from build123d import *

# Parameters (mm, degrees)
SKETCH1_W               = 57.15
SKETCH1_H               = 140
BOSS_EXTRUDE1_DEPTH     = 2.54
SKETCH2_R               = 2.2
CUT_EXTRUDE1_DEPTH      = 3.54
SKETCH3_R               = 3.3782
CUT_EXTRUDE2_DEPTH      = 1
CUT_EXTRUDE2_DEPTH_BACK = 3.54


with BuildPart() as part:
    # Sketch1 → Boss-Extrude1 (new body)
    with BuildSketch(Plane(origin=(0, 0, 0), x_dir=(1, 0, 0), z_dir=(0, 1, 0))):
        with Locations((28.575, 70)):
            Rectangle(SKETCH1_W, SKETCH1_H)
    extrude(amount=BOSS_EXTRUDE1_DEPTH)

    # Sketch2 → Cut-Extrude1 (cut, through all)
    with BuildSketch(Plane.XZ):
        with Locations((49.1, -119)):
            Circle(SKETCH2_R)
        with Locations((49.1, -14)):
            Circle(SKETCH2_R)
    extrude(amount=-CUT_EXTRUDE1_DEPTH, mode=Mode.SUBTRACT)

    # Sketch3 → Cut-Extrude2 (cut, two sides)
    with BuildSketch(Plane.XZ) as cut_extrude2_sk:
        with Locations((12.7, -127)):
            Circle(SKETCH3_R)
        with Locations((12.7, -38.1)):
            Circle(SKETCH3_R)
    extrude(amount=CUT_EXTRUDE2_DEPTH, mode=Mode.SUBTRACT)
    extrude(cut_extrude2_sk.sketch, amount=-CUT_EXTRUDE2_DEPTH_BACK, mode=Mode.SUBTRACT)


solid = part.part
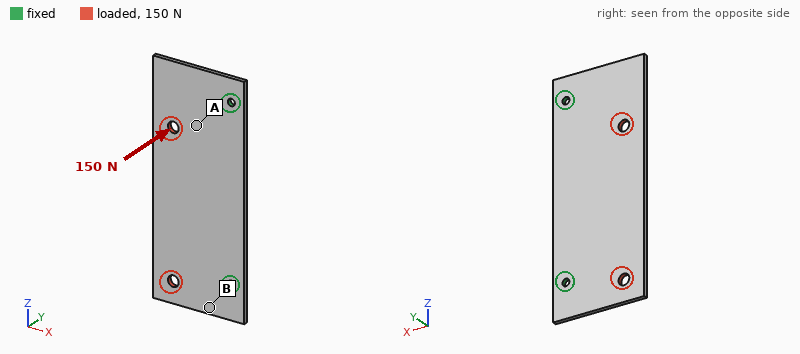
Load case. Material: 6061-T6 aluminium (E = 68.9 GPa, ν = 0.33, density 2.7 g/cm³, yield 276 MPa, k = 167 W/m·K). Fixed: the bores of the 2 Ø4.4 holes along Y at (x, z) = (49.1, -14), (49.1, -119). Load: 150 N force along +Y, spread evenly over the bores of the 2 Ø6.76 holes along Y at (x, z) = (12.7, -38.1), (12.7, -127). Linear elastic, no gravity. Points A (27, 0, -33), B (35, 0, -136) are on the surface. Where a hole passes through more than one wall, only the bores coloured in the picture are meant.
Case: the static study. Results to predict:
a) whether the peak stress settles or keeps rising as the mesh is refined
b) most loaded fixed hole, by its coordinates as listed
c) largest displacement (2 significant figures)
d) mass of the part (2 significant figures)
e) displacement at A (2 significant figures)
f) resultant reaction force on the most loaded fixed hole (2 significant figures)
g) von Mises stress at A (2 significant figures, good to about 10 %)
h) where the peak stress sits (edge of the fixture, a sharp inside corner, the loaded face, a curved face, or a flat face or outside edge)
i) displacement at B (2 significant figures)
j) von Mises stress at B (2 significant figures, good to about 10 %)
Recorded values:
keeps rising
(49.1, -119)
0.56 mm
54 g
0.20 mm
92 N
18 MPa
edge of the fixture
0.084 mm
36 MPa
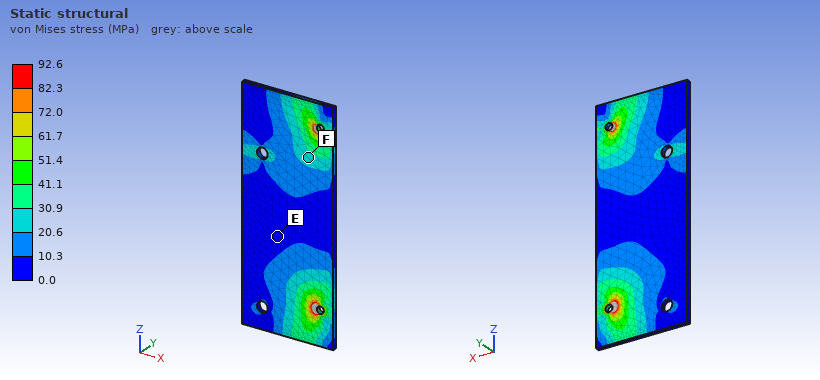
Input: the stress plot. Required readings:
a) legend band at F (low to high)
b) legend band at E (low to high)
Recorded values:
20.6 to 30.9 MPa
0.0 to 10.3 MPa
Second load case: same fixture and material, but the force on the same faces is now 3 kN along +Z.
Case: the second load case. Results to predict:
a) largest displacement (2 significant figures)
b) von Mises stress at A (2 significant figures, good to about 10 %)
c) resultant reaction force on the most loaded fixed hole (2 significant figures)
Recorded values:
42 µm
21 MPa
1.8 kN
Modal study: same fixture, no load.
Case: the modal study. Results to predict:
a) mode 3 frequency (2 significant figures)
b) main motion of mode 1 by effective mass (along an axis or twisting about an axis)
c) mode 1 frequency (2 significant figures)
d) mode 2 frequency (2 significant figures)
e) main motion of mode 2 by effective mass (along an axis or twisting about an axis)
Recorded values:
1200 Hz
along Y
570 Hz
1000 Hz
twisting about X
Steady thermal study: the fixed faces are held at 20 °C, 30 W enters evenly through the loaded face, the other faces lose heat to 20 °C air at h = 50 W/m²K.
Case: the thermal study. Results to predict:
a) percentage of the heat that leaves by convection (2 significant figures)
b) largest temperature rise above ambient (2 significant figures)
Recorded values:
40 %
35 K
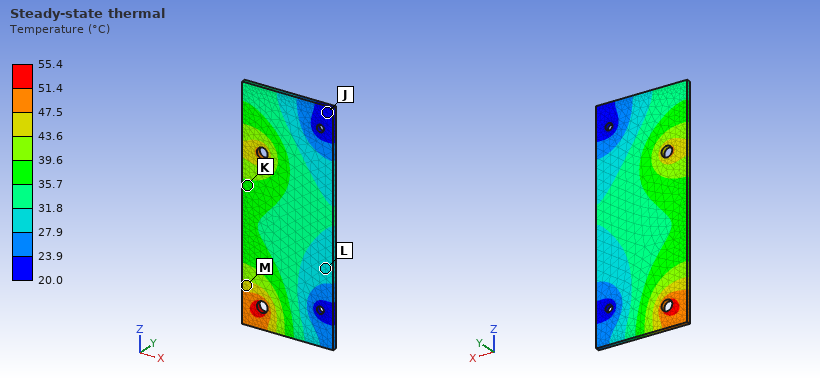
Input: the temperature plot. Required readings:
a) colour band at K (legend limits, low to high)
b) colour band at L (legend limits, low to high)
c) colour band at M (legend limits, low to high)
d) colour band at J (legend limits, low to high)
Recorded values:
35.7 to 39.6 °C
27.9 to 31.8 °C
43.6 to 47.5 °C
20.0 to 23.9 °C
